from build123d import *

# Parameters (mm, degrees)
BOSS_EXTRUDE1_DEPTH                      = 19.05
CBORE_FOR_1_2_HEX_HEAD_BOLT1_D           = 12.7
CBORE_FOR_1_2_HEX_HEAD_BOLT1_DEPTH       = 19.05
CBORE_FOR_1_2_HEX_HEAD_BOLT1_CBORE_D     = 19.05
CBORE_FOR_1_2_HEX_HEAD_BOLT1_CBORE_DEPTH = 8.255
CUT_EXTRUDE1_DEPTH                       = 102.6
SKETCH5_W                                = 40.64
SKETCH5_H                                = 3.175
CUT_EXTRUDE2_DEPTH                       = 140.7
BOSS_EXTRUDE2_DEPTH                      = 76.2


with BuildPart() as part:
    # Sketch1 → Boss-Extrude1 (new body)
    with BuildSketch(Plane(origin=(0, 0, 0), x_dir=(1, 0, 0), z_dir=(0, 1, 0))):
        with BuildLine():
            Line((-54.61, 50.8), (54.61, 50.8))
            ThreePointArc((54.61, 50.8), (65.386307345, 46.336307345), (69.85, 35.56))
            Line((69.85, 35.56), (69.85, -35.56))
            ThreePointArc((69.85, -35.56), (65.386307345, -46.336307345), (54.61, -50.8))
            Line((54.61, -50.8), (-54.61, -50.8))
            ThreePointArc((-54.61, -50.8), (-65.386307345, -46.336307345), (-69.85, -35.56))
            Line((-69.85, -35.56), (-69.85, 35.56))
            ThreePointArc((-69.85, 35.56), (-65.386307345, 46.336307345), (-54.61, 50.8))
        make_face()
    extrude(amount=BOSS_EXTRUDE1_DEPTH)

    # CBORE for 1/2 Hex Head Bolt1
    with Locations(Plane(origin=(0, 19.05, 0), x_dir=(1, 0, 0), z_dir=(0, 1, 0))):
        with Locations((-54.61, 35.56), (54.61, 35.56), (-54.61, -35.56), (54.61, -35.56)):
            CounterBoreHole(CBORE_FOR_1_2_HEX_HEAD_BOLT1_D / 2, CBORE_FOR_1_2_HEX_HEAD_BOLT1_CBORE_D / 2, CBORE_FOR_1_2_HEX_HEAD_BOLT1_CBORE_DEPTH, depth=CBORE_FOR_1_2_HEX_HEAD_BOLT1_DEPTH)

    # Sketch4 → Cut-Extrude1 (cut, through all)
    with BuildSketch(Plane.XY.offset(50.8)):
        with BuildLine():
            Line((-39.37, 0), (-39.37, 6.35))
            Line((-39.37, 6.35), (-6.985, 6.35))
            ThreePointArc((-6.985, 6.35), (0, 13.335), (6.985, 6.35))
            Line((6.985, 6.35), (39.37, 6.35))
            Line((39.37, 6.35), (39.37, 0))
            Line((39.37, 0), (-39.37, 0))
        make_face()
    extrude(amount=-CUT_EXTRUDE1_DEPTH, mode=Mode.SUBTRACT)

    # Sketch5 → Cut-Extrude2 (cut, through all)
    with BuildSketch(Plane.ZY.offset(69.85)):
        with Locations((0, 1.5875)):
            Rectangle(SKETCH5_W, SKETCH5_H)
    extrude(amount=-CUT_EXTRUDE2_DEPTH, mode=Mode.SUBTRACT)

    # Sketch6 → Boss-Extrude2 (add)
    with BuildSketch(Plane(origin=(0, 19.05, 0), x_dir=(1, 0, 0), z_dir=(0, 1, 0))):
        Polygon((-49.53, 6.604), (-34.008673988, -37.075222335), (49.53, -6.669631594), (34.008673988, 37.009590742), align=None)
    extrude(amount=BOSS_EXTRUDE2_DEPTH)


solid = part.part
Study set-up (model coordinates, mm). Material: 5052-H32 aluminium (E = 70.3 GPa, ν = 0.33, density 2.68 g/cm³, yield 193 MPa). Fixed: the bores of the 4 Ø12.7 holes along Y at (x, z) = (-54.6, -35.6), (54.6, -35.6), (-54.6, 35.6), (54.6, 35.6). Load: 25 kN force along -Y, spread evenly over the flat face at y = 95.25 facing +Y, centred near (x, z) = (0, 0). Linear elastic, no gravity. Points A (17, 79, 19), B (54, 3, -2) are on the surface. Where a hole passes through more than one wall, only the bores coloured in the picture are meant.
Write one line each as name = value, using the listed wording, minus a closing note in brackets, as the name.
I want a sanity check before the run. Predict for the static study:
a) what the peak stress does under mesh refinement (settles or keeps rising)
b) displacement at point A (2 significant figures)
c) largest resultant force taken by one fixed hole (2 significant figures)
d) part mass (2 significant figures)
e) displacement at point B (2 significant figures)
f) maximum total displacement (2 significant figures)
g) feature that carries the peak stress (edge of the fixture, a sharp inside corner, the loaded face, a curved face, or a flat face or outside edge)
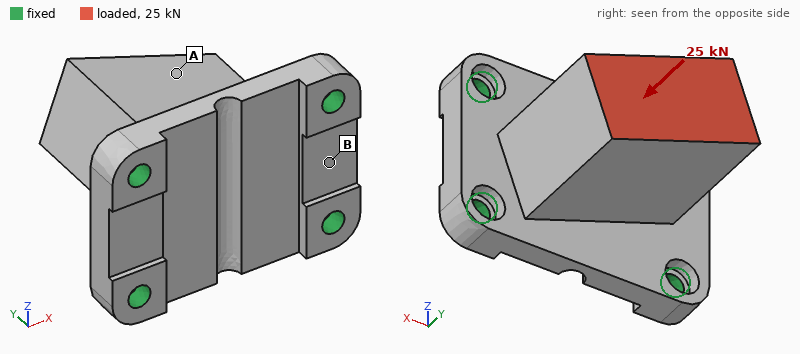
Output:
what the peak stress does under mesh refinement = keeps rising
displacement at point A = 32 µm
largest resultant force taken by one fixed hole = 11 kN
part mass = 1.3 kg
displacement at point B = 17 µm
maximum total displacement = 34 µm
feature that carries the peak stress = edge of the fixture
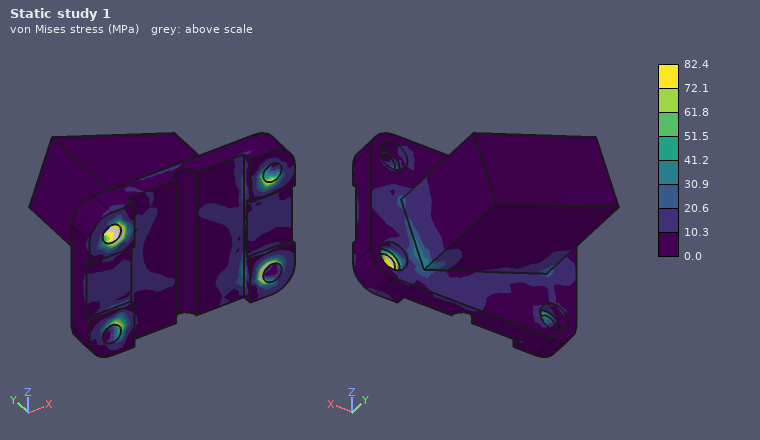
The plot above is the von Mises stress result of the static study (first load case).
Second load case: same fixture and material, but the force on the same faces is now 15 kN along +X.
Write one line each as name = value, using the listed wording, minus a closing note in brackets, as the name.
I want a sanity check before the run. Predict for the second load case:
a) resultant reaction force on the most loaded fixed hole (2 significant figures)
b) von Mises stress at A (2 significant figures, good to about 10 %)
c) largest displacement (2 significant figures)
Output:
resultant reaction force on the most loaded fixed hole = 9.3 kN
von Mises stress at A = 9.9 MPa
largest displacement = 0.11 mm
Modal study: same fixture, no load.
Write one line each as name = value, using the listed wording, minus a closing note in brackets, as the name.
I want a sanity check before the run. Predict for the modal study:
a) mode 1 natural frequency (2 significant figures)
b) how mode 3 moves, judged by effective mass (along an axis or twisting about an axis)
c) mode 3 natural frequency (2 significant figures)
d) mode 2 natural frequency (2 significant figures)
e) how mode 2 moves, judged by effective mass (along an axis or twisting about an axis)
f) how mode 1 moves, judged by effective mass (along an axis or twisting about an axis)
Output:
mode 1 natural frequency = 2300 Hz
how mode 3 moves, judged by effective mass = along Y
mode 3 natural frequency = 4500 Hz
mode 2 natural frequency = 3900 Hz
how mode 2 moves, judged by effective mass = along X
how mode 1 moves, judged by effective mass = along Z
